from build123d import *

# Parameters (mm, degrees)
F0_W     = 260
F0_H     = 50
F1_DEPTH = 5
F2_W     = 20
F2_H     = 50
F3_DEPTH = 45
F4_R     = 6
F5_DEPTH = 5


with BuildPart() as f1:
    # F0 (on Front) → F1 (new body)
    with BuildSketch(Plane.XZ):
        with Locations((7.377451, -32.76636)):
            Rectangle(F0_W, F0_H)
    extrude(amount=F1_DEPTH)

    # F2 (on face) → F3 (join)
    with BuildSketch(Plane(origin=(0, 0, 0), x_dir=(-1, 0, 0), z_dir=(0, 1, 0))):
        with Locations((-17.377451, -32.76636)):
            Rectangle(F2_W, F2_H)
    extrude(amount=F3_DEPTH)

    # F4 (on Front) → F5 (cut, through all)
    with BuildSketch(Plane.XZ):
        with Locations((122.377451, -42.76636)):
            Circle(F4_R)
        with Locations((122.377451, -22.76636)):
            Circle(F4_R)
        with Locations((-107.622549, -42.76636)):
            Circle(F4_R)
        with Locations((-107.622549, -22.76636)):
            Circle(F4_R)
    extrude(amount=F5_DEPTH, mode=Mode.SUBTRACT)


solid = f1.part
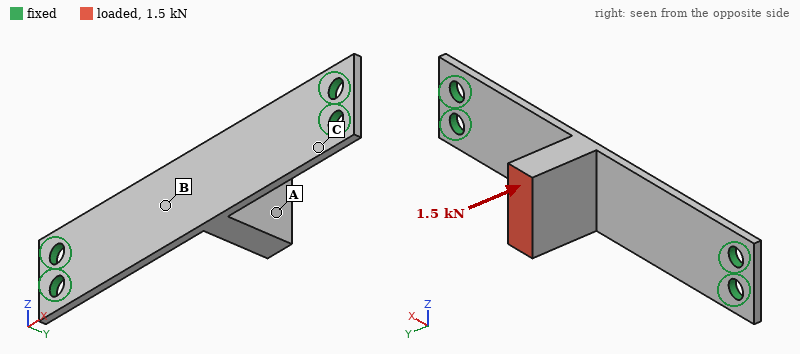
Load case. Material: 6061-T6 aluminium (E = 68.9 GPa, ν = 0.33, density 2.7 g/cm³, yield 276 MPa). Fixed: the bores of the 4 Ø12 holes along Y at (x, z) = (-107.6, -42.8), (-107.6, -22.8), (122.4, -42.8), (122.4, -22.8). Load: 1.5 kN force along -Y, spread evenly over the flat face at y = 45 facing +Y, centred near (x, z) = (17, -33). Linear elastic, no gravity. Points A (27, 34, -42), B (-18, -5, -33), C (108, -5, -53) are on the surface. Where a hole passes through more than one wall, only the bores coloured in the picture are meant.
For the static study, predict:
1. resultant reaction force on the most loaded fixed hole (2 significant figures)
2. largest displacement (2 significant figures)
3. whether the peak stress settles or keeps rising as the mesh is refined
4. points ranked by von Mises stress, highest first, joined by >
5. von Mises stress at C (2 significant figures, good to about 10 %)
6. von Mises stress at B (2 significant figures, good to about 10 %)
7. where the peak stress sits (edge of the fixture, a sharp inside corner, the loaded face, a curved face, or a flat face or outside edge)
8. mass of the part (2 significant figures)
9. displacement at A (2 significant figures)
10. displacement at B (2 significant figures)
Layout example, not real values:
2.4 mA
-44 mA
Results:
470 N
1.8 mm
keeps rising
C > B > A
140 MPa
86 MPa
edge of the fixture
290 g
1.7 mm
1.6 mm
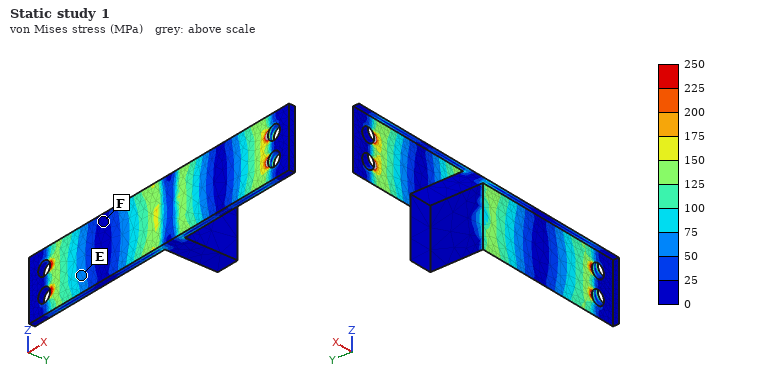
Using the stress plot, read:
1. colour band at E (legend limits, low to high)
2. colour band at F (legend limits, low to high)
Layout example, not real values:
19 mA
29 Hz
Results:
50 to 75 MPa
0 to 25 MPa
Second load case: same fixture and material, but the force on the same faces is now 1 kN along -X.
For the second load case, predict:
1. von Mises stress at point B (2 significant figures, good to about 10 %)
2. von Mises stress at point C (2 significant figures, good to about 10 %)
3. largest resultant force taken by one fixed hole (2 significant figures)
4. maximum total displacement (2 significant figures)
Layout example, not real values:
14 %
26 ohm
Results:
57 MPa
29 MPa
310 N
0.71 mm
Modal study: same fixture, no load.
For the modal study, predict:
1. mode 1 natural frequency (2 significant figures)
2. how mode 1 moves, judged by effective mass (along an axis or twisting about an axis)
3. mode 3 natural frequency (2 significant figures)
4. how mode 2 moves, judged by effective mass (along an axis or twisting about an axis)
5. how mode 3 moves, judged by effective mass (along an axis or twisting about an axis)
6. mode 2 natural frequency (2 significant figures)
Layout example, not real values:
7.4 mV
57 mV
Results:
340 Hz
along Y
840 Hz
along Z
along X
480 Hz
